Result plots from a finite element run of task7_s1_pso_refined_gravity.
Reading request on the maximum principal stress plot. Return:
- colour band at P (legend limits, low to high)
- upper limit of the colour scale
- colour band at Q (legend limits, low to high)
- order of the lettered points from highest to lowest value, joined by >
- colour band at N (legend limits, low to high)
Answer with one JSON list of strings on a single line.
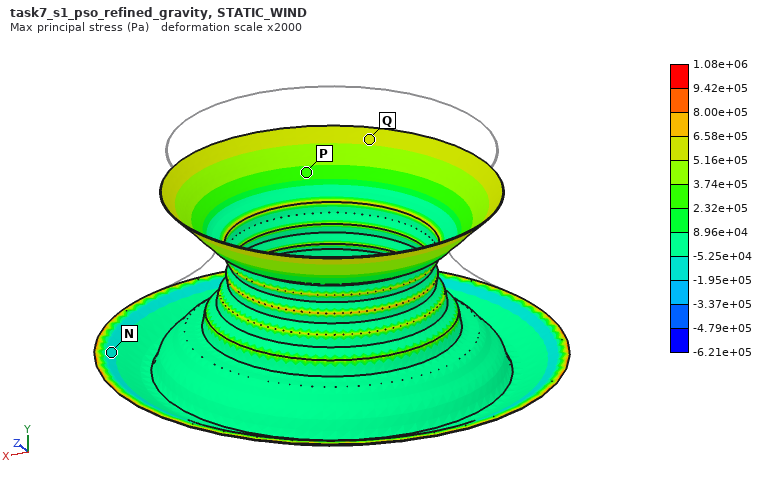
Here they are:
["2.32e+05 to 3.74e+05 Pa", "1.08e+06 Pa", "5.16e+05 to 6.58e+05 Pa", "Q > P > N", "-1.95e+05 to -5.25e+04 Pa"]
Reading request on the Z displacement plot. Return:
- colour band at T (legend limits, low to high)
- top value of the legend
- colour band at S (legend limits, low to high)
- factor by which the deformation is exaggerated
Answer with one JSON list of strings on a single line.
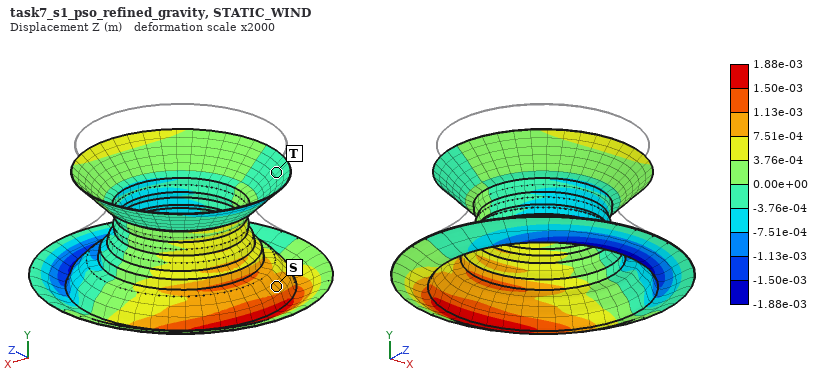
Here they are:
["-3.76e-04 to 0.00e+00 m", "1.88e-03 m", "7.51e-04 to 1.13e-03 m", "2000"]
